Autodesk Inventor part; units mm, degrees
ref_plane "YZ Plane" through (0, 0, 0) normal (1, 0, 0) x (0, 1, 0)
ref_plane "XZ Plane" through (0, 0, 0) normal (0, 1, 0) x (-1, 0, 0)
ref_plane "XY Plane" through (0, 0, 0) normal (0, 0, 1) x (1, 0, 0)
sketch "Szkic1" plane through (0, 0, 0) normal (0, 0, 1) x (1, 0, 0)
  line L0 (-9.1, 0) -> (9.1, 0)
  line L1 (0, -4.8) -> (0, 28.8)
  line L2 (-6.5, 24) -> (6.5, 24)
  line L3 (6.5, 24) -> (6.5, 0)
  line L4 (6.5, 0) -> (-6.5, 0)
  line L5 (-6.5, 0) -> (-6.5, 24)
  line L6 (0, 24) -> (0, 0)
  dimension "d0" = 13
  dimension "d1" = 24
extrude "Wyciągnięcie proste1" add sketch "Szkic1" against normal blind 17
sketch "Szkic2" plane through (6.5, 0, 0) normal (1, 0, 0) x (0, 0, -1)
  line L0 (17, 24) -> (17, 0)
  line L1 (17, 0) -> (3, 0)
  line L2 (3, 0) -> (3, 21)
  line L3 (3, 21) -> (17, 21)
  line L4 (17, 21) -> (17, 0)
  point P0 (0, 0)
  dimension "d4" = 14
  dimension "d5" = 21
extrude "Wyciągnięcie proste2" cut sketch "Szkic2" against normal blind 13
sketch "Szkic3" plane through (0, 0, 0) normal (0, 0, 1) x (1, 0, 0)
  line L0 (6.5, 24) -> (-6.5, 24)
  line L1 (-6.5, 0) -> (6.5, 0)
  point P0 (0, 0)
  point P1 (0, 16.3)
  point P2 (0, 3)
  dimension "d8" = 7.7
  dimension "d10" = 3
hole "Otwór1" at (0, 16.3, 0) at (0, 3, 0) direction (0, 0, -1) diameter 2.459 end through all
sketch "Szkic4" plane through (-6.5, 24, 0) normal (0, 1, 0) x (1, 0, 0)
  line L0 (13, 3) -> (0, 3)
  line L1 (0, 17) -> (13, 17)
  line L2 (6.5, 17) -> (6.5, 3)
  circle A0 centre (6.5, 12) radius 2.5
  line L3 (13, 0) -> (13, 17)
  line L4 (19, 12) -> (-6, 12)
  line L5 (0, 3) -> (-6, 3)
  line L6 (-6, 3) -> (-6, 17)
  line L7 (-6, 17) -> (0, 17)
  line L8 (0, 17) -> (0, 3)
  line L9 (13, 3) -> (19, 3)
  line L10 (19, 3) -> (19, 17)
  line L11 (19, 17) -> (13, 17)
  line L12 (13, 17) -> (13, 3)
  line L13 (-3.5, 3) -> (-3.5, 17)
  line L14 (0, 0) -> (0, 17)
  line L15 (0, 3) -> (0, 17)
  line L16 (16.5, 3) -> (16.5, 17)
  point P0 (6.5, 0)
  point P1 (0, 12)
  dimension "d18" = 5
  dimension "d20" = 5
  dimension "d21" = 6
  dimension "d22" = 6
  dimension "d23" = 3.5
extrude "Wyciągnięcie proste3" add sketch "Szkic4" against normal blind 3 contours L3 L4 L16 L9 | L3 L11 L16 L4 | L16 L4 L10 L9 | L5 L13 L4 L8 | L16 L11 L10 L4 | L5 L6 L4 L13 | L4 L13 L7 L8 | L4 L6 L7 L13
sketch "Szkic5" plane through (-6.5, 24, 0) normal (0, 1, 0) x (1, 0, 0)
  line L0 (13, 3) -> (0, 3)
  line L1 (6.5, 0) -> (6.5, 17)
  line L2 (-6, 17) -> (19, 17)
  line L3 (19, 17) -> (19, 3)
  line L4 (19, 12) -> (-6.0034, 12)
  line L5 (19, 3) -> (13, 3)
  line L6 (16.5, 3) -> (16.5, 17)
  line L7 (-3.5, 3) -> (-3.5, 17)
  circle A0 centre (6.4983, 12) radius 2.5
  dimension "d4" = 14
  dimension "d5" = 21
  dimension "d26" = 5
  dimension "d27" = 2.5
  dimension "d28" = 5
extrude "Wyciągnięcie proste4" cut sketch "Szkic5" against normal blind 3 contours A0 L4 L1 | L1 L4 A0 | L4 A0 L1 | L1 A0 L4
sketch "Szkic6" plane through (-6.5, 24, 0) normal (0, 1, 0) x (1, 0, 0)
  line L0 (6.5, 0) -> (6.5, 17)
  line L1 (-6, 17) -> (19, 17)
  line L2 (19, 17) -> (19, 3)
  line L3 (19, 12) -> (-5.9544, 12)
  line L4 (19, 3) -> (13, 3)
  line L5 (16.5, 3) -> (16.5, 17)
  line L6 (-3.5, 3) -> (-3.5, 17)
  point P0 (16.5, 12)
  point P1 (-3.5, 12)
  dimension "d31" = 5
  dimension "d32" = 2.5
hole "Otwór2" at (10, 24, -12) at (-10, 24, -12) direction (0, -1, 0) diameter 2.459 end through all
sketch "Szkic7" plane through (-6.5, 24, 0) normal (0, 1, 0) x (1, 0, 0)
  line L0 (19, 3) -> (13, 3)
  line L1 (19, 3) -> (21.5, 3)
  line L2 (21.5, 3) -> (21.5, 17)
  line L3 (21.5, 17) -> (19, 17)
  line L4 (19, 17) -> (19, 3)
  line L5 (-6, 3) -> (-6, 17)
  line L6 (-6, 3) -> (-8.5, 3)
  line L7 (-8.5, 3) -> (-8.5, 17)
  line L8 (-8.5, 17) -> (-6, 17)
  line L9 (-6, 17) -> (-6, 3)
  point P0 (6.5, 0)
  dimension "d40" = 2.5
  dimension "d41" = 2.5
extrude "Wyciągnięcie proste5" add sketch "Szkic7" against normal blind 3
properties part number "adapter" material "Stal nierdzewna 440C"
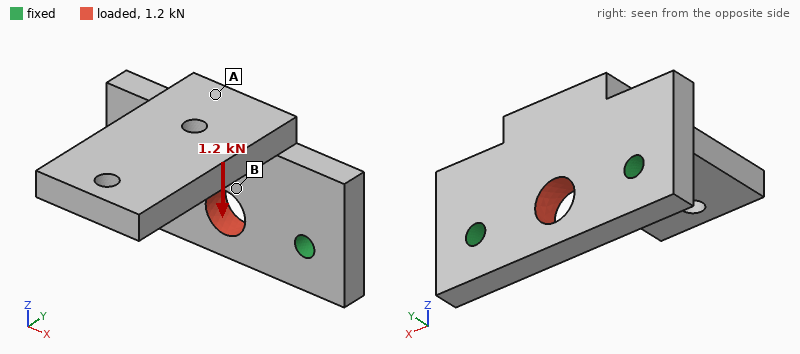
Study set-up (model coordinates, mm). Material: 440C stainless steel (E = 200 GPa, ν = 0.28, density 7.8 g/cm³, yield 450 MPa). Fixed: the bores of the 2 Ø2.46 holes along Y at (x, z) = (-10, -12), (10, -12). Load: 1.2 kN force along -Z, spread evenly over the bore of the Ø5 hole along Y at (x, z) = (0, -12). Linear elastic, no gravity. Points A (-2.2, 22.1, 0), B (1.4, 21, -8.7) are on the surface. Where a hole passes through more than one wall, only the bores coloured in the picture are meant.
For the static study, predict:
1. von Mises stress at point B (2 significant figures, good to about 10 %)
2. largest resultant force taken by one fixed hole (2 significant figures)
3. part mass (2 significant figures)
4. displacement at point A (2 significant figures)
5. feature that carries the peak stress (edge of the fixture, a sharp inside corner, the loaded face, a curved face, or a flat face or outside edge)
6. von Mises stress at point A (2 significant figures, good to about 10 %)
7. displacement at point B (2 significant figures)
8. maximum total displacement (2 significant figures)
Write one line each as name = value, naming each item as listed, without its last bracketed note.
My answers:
von Mises stress at point B = 27 MPa
largest resultant force taken by one fixed hole = 610 N
part mass = 16 g
displacement at point A = 1.6 µm
feature that carries the peak stress = edge of the fixture
von Mises stress at point A = 12 MPa
displacement at point B = 2.1 µm
maximum total displacement = 3.4 µm
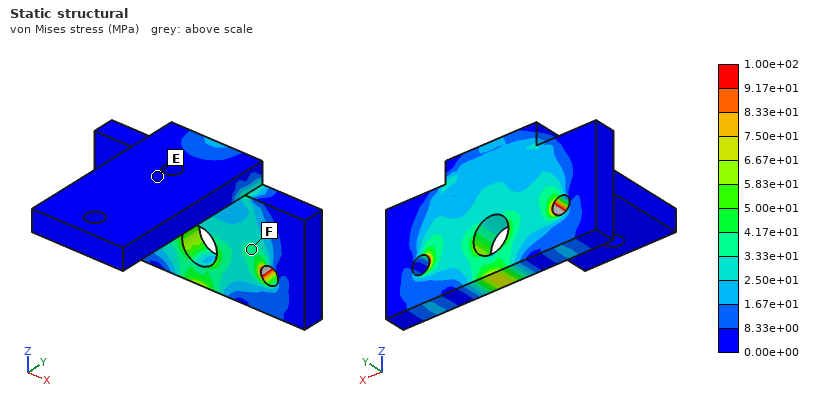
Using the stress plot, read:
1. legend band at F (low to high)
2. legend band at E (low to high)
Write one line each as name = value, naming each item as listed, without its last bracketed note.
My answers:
legend band at F = 3.33e+01 to 4.17e+01 MPa
legend band at E = 0.00e+00 to 8.33e+00 MPa
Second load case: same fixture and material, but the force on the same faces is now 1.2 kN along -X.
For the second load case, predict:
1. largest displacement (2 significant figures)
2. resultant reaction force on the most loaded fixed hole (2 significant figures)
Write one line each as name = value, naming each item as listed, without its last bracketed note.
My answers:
largest displacement = 1.2 µm
resultant reaction force on the most loaded fixed hole = 600 N
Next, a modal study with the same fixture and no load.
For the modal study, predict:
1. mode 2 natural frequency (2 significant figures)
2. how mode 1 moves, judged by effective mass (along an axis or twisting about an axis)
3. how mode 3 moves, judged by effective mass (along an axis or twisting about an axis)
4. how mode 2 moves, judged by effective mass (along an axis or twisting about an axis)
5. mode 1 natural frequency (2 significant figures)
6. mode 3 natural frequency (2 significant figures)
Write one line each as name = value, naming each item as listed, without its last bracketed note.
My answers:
mode 2 natural frequency = 6800 Hz
how mode 1 moves, judged by effective mass = along Z
how mode 3 moves, judged by effective mass = along Y
how mode 2 moves, judged by effective mass = along X
mode 1 natural frequency = 3100 Hz
mode 3 natural frequency = 9900 Hz
